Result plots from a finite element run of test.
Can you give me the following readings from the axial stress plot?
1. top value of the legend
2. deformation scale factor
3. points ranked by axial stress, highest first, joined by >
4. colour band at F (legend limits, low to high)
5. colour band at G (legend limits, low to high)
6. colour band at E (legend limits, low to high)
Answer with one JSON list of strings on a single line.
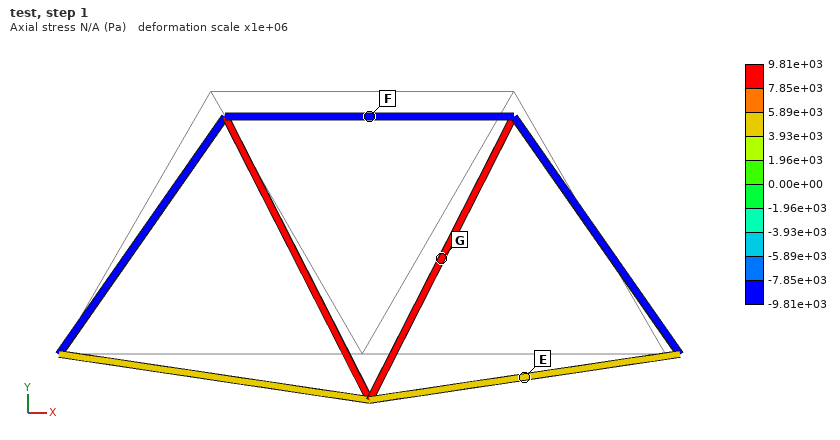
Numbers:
["9.81e+03 Pa", "1e+06", "G > E > F", "-9.81e+03 to -7.85e+03 Pa", "7.85e+03 to 9.81e+03 Pa", "3.93e+03 to 5.89e+03 Pa"]
